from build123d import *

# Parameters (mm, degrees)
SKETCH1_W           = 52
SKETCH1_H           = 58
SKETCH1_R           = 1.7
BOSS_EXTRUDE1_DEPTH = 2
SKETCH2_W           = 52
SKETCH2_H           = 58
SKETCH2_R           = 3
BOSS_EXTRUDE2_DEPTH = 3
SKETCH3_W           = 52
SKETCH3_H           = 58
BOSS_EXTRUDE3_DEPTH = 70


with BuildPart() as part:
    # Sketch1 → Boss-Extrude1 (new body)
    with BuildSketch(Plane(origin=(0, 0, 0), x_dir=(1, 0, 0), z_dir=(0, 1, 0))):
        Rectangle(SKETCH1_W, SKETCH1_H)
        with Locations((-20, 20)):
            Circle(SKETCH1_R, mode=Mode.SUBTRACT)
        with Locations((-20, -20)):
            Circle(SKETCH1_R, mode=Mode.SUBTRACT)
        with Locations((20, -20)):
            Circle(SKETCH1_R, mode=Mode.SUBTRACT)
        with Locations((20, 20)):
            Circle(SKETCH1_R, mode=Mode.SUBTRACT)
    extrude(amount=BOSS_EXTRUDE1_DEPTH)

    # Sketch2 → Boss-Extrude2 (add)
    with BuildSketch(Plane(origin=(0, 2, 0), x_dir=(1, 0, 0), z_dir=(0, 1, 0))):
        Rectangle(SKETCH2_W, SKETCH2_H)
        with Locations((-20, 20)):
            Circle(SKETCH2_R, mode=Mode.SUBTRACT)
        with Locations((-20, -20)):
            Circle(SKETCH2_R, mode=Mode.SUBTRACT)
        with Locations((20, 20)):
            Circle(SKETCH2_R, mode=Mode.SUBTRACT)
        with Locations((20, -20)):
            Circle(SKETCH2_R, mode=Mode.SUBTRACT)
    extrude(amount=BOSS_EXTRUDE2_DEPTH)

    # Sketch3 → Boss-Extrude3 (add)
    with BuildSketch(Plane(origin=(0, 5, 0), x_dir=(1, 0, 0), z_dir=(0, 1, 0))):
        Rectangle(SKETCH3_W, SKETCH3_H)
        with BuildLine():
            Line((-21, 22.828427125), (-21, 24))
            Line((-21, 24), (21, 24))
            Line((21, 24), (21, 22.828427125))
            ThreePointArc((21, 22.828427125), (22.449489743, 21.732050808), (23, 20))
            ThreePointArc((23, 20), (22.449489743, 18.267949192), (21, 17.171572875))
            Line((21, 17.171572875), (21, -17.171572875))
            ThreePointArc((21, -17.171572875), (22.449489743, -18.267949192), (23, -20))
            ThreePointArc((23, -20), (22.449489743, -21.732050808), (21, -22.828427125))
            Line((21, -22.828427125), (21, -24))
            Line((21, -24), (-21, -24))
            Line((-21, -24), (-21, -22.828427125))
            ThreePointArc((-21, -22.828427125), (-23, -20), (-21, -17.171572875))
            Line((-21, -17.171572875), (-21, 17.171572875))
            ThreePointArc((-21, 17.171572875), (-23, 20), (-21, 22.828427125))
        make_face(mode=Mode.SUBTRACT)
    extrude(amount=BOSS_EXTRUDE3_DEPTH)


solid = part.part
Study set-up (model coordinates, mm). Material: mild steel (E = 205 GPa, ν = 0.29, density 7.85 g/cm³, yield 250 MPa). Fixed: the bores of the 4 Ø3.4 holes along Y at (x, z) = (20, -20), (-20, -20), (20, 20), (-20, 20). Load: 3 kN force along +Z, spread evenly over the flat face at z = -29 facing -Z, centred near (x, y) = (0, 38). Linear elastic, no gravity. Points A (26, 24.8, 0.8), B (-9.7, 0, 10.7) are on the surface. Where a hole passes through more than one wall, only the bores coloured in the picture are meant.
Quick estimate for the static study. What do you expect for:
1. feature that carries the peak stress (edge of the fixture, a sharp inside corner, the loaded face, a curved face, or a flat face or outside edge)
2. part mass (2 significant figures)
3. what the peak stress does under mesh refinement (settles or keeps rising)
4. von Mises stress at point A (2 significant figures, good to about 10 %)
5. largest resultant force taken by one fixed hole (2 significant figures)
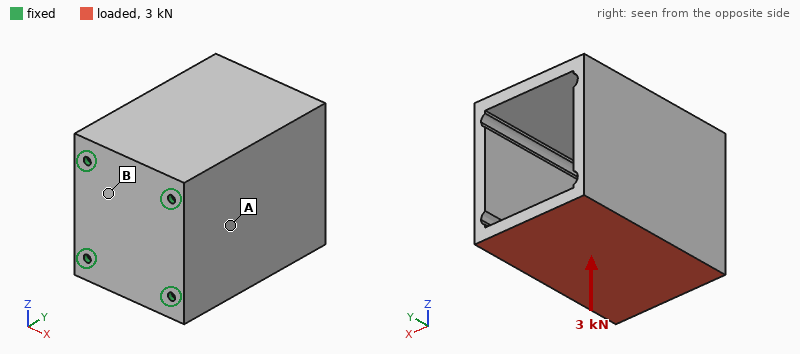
edge of the fixture
650 g
keeps rising
13 MPa
1.5 kN
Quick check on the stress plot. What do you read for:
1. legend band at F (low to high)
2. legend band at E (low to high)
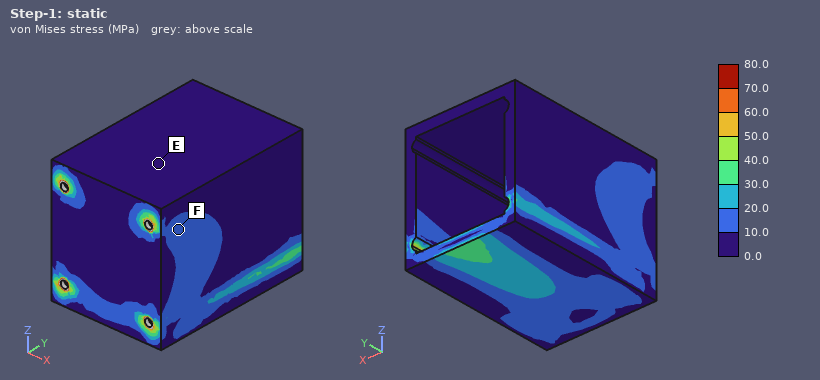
10.0 to 20.0 MPa
0.0 to 10.0 MPa
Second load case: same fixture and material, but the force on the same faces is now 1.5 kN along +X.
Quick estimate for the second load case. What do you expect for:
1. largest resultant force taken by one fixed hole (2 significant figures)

1.3 kN
